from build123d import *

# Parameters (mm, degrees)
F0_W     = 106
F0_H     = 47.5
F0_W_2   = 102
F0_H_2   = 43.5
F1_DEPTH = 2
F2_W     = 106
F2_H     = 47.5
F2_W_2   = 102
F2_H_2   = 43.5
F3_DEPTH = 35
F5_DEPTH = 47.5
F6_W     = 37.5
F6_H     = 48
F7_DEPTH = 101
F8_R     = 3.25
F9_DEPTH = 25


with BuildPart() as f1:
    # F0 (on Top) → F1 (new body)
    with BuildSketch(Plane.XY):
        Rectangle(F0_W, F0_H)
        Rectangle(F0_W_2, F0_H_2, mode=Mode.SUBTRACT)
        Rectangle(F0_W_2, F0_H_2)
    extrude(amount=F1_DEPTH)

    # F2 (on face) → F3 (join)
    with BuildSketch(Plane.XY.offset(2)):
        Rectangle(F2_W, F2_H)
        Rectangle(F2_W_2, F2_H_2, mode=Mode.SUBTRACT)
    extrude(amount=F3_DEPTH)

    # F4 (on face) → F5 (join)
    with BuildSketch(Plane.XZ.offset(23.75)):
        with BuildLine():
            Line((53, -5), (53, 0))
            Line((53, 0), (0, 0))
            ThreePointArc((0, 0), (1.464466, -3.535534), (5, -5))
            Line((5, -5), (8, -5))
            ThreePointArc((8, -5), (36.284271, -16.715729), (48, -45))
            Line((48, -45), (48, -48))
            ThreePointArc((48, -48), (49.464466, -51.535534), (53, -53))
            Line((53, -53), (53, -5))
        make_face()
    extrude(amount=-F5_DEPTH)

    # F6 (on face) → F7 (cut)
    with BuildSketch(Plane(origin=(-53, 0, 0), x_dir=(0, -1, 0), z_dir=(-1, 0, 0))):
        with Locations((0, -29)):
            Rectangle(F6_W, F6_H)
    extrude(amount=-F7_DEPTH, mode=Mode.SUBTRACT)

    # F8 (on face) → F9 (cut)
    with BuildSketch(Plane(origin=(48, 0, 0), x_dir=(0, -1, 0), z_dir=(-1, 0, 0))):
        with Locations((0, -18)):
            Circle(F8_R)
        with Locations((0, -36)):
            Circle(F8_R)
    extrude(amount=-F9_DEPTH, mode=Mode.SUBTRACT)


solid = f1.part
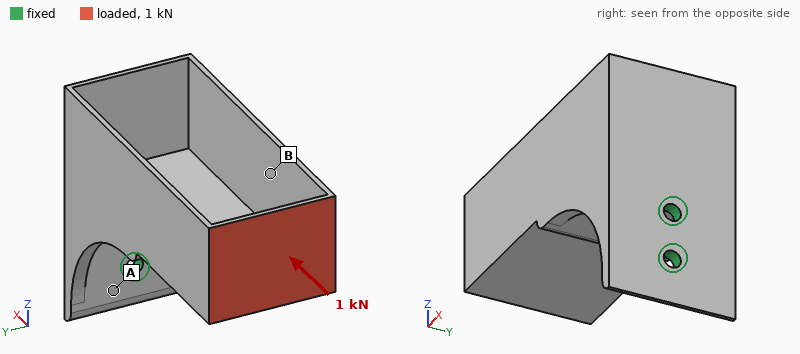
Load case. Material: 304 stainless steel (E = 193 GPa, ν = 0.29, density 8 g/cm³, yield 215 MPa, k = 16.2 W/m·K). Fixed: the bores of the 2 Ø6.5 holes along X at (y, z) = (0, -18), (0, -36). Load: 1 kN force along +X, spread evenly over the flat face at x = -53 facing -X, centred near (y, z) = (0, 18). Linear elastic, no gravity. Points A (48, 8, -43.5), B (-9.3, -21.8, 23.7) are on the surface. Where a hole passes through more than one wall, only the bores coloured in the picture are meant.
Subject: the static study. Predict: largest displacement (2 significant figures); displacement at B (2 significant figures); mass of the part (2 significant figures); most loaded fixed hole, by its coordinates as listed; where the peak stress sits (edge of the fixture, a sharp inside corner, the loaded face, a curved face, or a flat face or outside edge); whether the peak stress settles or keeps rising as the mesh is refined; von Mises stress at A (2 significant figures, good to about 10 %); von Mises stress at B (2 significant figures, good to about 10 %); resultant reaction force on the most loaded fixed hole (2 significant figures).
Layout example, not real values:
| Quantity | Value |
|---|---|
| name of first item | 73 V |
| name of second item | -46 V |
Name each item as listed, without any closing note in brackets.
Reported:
| Quantity | Value |
|---|---|
| largest displacement | 0.25 mm |
| displacement at B | 0.12 mm |
| mass of the part | 460 g |
| most loaded fixed hole, by its coordinates as listed | (0, -18) |
| where the peak stress sits | edge of the fixture |
| whether the peak stress settles or keeps rising as the mesh is refined | keeps rising |
| von Mises stress at A | 26 MPa |
| von Mises stress at B | 9.1 MPa |
| resultant reaction force on the most loaded fixed hole | 2.1 kN |
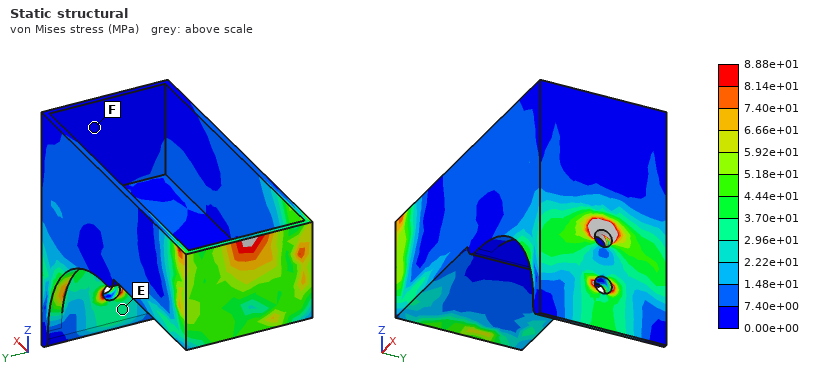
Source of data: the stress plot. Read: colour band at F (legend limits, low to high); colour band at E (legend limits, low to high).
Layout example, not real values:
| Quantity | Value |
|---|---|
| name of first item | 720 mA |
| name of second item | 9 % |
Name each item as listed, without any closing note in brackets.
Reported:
| Quantity | Value |
|---|---|
| colour band at F | 0.00e+00 to 7.40e+00 MPa |
| colour band at E | 2.96e+01 to 3.70e+01 MPa |
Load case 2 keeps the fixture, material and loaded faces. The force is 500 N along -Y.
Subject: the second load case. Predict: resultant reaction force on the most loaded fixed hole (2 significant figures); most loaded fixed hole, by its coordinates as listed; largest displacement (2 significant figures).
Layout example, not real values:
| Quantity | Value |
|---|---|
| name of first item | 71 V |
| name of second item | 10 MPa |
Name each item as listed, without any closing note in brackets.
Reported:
| Quantity | Value |
|---|---|
| resultant reaction force on the most loaded fixed hole | 1.2 kN |
| most loaded fixed hole, by its coordinates as listed | (0, -18) |
| largest displacement | 0.27 mm |
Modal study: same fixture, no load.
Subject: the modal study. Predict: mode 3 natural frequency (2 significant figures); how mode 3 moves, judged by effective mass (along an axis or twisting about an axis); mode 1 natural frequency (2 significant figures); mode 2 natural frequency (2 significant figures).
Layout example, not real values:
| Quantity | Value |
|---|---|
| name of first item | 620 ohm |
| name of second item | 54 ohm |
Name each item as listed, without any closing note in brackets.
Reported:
| Quantity | Value |
|---|---|
| mode 3 natural frequency | 1200 Hz |
| how mode 3 moves, judged by effective mass | twisting about X |
| mode 1 natural frequency | 640 Hz |
| mode 2 natural frequency | 670 Hz |
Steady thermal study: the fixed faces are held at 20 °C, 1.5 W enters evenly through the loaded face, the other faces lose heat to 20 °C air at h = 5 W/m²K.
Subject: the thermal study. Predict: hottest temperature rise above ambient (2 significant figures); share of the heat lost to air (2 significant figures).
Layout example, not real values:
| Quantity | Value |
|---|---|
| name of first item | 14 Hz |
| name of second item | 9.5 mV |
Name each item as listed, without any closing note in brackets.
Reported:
| Quantity | Value |
|---|---|
| hottest temperature rise above ambient | 23 K |
| share of the heat lost to air | 74 % |
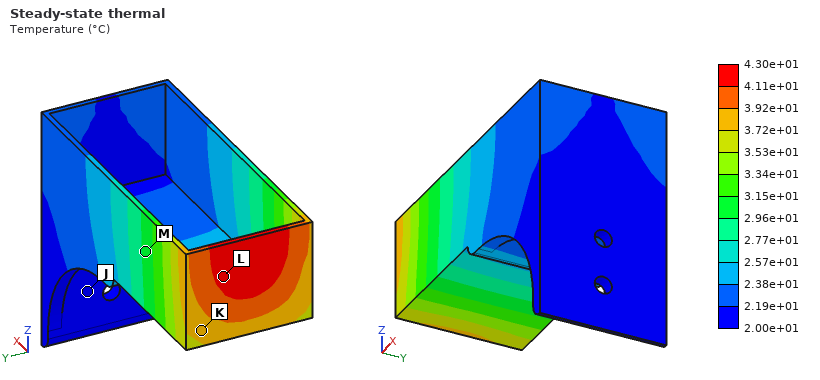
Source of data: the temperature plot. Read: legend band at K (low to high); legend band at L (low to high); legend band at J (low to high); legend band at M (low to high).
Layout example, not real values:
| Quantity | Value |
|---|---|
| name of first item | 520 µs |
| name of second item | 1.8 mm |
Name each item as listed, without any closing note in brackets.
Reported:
| Quantity | Value |
|---|---|
| legend band at K | 3.72e+01 to 3.92e+01 °C |
| legend band at L | 4.11e+01 to 4.30e+01 °C |
| legend band at J | 2.00e+01 to 2.19e+01 °C |
| legend band at M | 2.96e+01 to 3.15e+01 °C |
